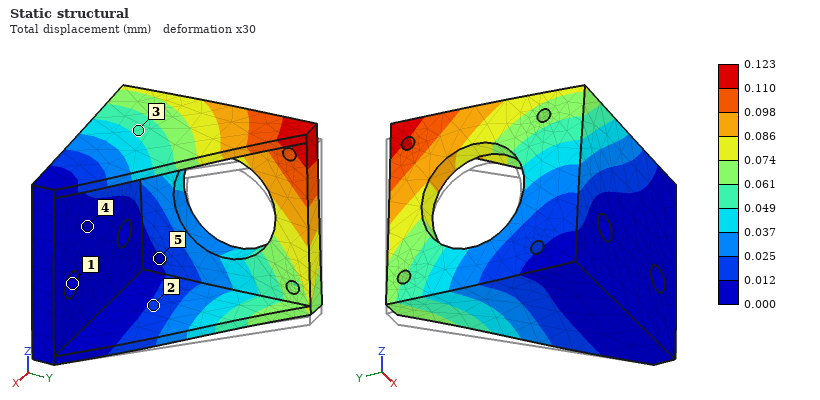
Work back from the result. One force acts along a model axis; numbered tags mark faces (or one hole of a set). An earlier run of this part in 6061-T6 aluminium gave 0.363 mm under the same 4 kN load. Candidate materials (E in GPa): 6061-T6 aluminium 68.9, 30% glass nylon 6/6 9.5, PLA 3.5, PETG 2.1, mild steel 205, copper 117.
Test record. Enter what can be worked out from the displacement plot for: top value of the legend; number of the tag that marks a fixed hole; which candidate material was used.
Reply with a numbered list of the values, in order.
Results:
1. 0.123 mm
2. 1
3. mild steel
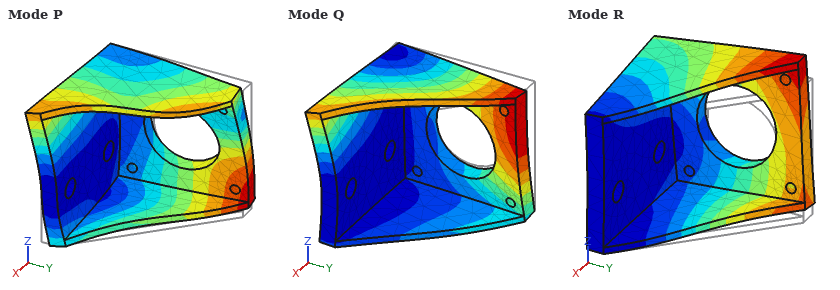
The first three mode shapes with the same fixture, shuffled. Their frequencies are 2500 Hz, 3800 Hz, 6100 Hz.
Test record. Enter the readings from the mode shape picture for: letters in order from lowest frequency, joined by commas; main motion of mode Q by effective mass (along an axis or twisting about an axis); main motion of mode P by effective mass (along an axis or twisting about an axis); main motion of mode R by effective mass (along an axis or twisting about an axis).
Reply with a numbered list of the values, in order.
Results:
1. R, Q, P
2. along X
3. along Y
4. along Z
